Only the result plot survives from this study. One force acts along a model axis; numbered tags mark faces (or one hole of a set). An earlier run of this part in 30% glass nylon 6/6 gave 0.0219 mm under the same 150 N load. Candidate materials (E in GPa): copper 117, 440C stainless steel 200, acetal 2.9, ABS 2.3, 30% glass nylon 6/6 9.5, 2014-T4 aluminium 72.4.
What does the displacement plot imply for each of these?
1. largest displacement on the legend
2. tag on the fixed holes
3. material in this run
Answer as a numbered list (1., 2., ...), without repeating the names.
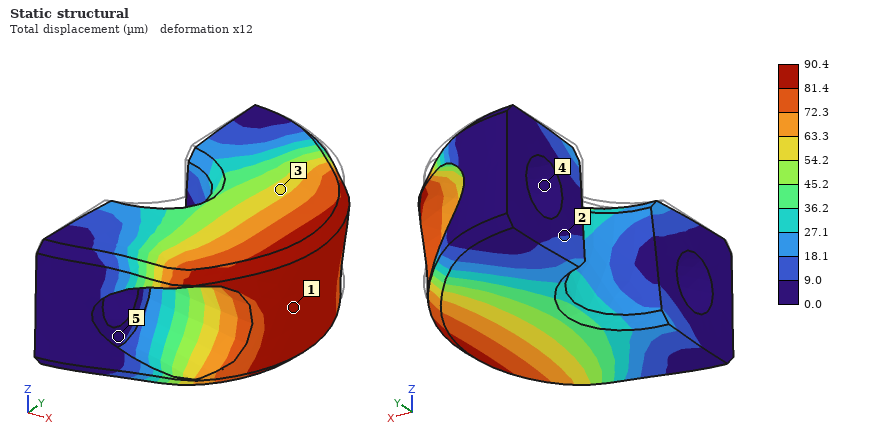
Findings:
1. 90.4 µm
2. 4
3. ABS
